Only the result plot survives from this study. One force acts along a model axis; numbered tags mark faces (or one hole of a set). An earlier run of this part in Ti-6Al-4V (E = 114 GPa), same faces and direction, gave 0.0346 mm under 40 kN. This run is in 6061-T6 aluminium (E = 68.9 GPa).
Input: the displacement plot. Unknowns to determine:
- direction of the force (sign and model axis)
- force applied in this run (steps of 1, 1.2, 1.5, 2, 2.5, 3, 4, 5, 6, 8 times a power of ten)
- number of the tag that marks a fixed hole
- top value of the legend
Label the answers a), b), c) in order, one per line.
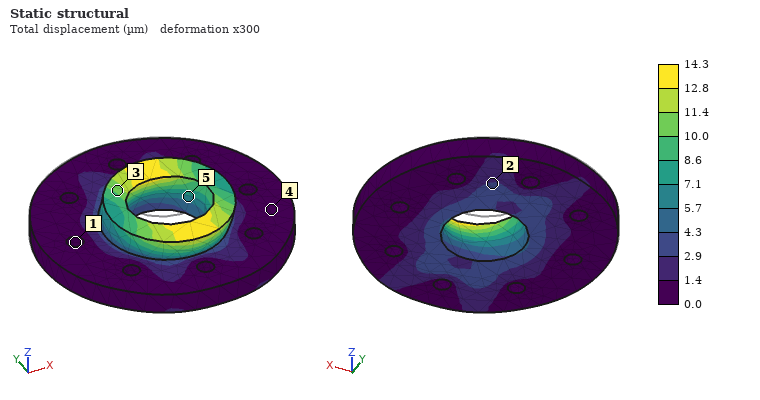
a) -Y
b) 10 kN
c) 1
d) 14.3 µm
